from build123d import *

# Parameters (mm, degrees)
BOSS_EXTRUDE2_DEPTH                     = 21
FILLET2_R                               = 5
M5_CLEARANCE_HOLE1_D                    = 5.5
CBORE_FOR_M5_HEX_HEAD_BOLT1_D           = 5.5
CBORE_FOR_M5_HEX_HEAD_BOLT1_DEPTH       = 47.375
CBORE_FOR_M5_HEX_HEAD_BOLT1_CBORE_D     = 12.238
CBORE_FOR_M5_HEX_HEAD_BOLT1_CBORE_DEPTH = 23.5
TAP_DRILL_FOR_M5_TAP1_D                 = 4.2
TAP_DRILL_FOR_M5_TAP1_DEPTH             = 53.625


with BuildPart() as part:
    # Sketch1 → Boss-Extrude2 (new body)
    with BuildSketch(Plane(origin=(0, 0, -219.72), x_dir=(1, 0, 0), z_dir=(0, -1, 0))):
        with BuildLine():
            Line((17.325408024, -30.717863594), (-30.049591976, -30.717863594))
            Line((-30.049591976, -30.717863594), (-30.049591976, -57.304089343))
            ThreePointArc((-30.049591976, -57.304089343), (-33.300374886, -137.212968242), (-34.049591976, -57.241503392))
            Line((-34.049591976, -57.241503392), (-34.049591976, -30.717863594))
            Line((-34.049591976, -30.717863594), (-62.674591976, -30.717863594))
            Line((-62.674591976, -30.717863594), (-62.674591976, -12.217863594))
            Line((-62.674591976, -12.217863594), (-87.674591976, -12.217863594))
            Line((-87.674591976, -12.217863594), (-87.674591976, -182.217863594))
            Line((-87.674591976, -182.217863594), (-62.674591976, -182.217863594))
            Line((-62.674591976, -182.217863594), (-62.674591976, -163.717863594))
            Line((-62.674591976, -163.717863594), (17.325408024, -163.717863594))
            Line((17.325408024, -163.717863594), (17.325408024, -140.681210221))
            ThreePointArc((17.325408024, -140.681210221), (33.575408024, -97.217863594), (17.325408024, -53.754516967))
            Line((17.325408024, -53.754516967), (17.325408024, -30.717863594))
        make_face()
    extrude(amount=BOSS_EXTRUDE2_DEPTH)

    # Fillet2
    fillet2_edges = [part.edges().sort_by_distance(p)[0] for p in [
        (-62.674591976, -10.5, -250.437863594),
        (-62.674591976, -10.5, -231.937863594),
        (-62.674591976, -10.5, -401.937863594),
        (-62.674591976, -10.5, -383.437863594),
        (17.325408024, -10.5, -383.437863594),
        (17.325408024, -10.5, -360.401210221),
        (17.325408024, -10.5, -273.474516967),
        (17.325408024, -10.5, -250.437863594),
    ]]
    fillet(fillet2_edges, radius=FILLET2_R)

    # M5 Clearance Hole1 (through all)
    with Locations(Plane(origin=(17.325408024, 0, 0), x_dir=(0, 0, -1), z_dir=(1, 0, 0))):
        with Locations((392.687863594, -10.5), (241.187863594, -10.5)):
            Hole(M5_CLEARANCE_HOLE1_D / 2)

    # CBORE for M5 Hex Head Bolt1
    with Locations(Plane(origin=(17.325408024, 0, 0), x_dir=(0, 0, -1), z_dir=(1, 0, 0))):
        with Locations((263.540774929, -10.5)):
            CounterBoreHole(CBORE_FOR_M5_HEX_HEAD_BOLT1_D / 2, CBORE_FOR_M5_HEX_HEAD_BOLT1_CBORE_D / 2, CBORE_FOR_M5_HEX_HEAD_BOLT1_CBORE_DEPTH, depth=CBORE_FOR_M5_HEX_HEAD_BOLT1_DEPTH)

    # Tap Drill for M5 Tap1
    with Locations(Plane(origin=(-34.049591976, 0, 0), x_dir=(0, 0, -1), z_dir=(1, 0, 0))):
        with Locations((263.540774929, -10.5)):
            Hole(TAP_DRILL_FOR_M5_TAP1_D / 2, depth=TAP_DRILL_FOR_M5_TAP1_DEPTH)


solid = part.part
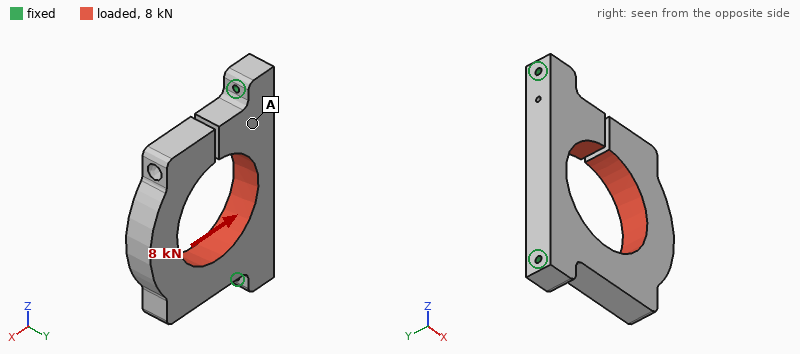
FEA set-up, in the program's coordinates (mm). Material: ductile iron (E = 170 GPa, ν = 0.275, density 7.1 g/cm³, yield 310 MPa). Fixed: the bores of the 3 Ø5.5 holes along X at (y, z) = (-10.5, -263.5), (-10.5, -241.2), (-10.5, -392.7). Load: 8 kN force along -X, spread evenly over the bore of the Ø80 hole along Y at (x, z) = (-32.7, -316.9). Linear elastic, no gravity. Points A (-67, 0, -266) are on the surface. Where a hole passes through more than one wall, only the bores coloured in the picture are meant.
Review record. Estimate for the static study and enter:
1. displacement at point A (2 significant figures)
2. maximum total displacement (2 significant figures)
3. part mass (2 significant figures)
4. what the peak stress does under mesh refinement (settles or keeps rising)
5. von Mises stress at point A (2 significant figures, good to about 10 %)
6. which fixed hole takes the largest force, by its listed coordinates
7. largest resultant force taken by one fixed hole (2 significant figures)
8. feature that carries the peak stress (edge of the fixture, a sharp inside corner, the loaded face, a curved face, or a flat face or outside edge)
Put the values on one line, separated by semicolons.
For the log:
5.4 µm; 14 µm; 1.6 kg; keeps rising; 8.1 MPa; (-10.5, -392.7); 4.2 kN; edge of the fixture
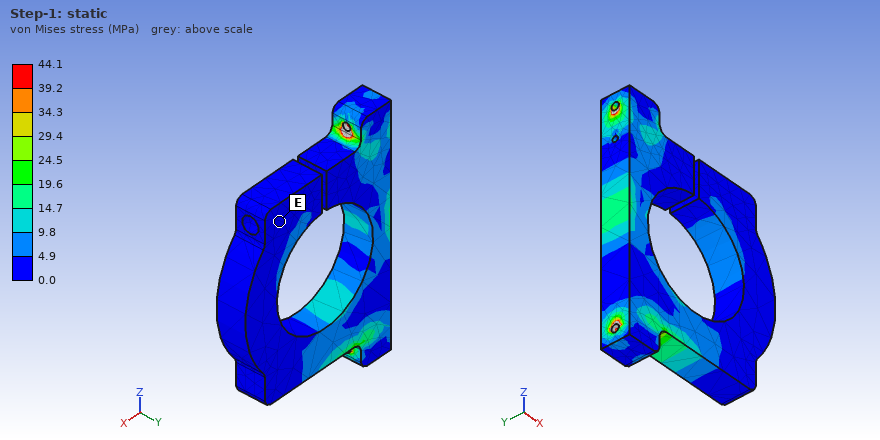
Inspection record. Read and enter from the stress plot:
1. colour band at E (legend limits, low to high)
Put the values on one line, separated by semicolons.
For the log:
0.0 to 4.9 MPa
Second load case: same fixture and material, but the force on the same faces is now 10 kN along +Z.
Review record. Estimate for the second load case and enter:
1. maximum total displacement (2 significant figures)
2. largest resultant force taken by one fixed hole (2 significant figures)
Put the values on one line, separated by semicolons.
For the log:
7.8 µm; 3.9 kN
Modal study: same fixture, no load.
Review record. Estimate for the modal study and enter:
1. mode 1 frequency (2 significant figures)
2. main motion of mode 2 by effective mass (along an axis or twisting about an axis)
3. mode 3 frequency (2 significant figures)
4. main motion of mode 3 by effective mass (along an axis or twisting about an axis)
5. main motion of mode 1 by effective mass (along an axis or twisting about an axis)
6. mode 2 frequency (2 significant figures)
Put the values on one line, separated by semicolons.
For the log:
1600 Hz; along Y; 4200 Hz; along X; along Y; 3200 Hz
